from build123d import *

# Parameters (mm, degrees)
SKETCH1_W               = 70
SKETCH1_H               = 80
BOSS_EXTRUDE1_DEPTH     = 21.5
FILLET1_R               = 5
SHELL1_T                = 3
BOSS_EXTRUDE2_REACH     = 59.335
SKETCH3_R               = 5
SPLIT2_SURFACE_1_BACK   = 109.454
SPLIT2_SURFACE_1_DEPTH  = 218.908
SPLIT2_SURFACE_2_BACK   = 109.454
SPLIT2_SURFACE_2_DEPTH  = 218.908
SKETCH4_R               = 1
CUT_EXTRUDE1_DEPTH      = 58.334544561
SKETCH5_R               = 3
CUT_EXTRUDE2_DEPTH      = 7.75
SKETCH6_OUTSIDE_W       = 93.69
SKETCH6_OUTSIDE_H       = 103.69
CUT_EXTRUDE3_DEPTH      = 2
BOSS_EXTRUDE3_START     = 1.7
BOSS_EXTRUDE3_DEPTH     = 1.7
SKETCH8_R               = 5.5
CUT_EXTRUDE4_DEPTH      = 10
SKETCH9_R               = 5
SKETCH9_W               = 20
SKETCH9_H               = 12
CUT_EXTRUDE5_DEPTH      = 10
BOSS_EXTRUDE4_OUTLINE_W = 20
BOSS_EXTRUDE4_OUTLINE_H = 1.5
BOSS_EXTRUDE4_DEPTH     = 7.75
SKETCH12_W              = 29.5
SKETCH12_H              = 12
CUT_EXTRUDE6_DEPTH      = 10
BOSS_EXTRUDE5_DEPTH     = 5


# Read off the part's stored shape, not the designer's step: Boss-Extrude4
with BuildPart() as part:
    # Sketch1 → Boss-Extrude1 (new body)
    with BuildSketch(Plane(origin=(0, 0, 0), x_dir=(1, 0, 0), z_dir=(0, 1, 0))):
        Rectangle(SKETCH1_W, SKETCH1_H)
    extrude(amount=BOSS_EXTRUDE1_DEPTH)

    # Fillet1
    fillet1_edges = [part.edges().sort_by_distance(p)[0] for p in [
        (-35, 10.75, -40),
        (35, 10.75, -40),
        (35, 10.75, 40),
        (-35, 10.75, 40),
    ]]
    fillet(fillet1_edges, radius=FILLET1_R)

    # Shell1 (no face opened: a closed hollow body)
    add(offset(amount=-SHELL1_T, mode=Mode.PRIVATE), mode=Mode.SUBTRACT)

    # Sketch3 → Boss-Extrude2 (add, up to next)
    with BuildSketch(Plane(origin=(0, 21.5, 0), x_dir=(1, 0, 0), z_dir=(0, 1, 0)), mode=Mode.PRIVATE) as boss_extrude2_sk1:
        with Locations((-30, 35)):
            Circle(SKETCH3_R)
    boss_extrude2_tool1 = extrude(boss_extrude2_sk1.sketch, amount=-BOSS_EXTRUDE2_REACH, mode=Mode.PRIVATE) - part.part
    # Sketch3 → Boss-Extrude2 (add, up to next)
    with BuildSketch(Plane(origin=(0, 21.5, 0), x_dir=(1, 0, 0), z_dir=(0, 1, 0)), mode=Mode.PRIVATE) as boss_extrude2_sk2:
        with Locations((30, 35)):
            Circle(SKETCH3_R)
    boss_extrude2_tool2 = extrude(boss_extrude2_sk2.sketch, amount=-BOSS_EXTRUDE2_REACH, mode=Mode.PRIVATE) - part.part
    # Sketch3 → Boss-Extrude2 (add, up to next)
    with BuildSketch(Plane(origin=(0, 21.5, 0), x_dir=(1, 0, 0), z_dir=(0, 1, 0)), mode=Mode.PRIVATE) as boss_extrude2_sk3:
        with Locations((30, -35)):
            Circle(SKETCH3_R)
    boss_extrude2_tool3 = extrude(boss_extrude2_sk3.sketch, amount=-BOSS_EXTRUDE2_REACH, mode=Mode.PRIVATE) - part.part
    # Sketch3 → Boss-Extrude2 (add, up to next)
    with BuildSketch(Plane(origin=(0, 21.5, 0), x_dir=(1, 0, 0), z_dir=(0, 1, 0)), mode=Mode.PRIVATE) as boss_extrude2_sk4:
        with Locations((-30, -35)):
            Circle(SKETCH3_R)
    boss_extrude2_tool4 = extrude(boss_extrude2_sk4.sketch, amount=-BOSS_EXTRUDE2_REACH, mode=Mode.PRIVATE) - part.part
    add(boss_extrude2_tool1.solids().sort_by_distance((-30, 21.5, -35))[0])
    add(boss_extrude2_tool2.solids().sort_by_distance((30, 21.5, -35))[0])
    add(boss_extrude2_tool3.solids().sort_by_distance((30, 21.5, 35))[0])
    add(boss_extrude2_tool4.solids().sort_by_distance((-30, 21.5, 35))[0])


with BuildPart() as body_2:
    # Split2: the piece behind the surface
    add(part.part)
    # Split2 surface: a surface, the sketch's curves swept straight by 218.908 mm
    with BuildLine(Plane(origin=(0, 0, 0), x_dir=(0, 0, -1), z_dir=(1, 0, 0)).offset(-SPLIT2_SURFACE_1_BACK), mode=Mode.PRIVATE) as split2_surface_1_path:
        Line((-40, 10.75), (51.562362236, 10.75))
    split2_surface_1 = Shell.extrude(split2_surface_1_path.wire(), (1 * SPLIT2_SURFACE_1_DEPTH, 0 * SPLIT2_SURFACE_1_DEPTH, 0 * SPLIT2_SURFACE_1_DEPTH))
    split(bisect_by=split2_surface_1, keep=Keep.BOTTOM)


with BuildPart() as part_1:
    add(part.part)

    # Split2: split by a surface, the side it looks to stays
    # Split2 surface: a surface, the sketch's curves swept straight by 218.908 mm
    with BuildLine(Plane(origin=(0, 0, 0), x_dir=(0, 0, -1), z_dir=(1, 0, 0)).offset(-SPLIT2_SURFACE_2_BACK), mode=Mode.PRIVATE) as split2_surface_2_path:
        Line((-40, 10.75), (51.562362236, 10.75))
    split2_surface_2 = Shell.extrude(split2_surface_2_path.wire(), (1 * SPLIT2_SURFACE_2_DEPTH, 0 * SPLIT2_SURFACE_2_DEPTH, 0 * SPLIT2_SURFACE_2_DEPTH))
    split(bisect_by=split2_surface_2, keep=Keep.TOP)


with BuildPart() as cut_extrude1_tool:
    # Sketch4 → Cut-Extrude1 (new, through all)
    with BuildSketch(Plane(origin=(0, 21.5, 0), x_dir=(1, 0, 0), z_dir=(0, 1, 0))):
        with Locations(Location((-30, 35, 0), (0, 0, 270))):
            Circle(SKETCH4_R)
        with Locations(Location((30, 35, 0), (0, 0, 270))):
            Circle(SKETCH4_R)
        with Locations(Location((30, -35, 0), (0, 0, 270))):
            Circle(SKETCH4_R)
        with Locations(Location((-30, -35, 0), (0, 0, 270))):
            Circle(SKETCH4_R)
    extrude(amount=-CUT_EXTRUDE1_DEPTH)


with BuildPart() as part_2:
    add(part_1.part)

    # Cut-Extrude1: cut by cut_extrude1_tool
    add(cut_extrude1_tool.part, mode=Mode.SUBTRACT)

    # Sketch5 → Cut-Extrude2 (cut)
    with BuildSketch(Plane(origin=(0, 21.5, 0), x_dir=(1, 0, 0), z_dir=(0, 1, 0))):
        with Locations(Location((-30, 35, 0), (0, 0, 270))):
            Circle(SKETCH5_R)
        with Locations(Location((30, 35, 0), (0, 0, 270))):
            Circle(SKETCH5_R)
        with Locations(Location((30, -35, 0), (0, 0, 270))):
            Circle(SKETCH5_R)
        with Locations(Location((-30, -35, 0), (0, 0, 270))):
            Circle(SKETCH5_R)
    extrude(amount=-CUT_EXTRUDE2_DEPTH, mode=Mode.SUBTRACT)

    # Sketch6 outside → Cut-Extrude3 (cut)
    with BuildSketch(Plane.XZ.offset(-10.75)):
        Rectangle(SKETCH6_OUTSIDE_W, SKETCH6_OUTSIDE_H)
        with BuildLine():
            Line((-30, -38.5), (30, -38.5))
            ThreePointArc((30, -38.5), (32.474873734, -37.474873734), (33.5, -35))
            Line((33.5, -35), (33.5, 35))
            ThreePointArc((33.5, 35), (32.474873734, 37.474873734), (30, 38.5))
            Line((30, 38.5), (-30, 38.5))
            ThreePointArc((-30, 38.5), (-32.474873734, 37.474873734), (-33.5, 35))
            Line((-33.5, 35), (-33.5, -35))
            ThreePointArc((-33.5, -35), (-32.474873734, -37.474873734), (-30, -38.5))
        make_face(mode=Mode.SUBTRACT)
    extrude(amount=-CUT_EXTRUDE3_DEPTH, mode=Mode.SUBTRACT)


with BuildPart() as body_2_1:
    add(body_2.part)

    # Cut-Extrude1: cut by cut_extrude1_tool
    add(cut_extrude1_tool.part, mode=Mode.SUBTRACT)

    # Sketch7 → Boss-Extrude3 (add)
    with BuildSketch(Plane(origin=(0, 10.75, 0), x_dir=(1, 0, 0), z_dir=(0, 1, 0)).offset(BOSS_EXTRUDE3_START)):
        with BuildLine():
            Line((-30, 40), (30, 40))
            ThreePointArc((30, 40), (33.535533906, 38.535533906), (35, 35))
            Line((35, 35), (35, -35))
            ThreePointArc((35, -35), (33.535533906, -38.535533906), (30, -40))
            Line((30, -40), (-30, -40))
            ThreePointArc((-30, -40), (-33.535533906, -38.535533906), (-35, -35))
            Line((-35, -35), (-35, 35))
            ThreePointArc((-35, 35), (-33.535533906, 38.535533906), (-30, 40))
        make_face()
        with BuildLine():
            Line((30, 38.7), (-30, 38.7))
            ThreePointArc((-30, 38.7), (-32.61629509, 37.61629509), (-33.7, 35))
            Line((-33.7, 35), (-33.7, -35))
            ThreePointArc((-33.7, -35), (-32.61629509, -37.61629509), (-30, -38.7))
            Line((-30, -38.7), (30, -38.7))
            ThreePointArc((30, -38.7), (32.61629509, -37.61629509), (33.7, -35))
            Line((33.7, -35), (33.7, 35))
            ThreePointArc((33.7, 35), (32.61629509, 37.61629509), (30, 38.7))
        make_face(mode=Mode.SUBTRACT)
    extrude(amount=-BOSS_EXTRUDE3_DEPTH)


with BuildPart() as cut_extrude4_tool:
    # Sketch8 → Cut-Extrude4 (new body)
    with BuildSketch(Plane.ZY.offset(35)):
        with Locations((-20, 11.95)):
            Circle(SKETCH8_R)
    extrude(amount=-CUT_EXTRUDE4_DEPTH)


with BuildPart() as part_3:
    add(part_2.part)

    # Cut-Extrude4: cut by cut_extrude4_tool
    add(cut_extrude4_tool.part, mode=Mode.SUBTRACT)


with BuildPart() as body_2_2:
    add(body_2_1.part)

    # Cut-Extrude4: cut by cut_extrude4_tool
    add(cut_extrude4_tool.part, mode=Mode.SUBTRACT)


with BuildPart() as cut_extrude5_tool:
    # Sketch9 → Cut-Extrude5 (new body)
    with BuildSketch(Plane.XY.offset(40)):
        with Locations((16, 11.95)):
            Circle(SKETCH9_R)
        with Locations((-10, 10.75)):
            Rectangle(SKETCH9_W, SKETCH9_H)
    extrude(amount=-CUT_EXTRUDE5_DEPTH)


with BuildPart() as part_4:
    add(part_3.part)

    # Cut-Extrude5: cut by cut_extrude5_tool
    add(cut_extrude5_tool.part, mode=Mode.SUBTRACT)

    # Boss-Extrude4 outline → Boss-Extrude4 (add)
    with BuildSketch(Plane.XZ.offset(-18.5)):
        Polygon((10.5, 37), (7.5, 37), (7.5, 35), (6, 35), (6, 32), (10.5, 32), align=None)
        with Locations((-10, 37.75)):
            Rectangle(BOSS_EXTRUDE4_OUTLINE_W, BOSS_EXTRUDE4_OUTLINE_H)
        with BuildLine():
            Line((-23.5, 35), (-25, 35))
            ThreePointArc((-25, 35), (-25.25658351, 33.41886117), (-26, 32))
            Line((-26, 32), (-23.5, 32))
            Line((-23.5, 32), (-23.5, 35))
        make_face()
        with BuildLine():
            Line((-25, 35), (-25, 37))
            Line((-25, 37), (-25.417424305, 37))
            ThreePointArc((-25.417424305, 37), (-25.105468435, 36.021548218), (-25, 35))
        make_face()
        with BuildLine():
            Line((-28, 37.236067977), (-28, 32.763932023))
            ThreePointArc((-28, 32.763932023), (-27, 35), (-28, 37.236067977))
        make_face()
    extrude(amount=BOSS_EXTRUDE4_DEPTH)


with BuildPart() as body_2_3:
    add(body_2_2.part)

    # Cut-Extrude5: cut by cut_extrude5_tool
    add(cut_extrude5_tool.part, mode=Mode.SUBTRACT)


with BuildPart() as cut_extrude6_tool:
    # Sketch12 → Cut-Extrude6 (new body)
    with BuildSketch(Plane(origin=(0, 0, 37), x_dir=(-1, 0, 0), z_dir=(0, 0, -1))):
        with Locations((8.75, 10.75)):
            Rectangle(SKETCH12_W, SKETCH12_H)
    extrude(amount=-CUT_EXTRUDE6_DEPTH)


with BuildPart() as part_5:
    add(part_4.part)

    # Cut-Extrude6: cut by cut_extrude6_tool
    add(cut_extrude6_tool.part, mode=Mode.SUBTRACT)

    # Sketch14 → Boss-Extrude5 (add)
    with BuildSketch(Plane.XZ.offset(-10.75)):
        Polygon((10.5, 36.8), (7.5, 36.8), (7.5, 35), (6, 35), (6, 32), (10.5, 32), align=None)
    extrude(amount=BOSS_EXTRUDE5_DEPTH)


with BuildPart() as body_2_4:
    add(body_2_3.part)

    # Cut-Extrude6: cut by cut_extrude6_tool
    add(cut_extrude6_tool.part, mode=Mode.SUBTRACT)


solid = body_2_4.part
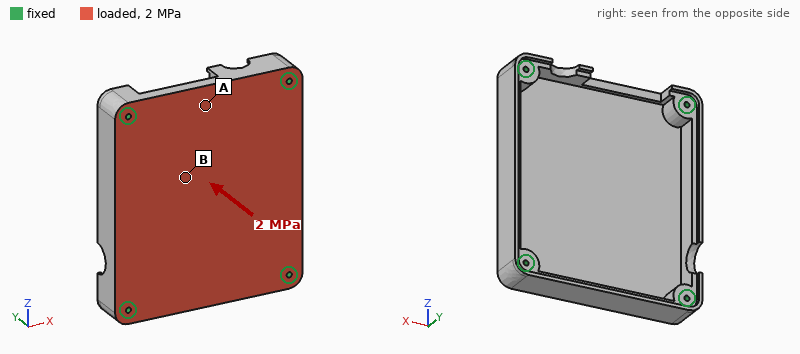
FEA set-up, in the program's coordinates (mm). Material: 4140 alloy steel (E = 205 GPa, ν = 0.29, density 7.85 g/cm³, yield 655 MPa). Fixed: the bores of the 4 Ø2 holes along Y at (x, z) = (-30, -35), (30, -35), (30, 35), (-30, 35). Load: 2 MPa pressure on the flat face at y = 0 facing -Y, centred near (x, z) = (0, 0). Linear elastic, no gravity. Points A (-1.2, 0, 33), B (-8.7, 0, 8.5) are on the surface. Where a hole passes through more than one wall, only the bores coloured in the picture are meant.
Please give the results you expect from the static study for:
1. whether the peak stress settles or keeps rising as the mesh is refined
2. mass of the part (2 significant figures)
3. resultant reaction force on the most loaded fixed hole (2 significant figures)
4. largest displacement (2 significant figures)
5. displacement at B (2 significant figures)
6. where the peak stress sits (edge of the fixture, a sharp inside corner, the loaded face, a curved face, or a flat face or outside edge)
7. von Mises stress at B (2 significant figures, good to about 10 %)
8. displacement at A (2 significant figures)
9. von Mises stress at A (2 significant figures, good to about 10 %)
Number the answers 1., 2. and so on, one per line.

1. keeps rising
2. 190 g
3. 3.5 kN
4. 0.28 mm
5. 0.24 mm
6. edge of the fixture
7. 210 MPa
8. 0.097 mm
9. 150 MPa
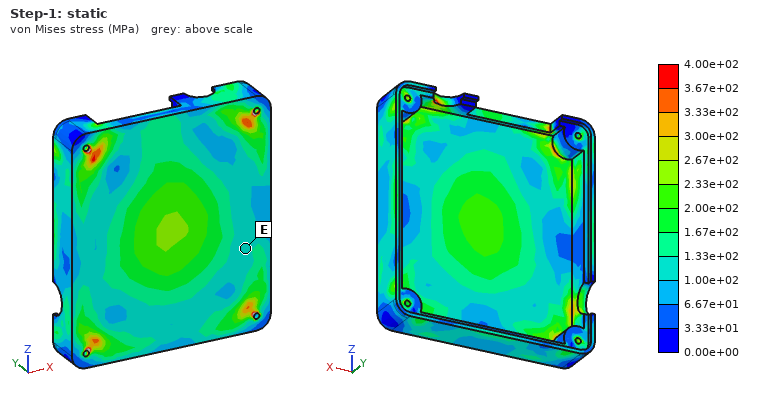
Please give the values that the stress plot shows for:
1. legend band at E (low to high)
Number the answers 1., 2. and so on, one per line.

1. 1.00e+02 to 1.33e+02 MPa
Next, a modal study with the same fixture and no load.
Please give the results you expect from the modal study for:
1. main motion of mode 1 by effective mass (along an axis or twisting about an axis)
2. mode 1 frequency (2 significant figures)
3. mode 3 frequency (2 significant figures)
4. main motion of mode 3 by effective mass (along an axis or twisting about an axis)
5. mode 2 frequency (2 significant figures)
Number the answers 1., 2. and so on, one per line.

1. along Y
2. 3500 Hz
3. 7200 Hz
4. twisting about Z
5. 6800 Hz
